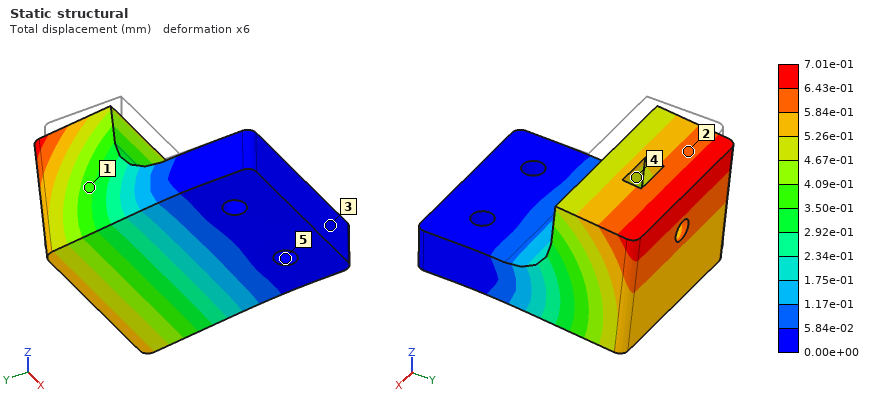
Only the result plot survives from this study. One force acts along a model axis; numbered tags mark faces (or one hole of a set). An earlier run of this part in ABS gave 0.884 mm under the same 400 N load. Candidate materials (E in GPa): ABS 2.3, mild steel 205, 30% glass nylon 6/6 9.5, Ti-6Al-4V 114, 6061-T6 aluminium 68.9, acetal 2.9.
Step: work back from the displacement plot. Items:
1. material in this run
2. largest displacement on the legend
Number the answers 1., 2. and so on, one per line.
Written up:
1. acetal
2. 7.01e-01 mm
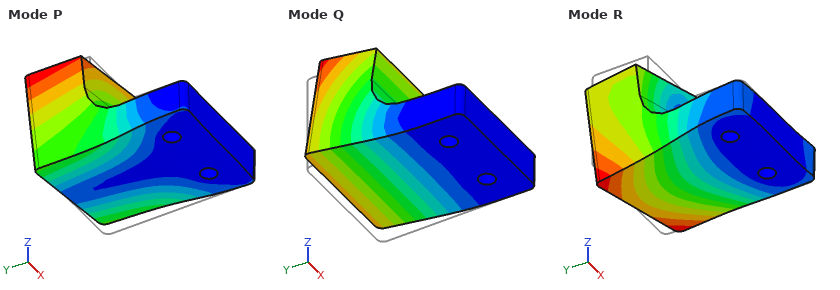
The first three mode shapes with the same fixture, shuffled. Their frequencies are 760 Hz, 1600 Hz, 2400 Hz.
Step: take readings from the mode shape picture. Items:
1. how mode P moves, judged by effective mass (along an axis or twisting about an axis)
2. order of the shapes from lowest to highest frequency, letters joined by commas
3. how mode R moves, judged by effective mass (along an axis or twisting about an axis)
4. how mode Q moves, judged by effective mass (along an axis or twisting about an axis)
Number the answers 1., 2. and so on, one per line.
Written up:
1. along X
2. Q, P, R
3. along X
4. along Z
